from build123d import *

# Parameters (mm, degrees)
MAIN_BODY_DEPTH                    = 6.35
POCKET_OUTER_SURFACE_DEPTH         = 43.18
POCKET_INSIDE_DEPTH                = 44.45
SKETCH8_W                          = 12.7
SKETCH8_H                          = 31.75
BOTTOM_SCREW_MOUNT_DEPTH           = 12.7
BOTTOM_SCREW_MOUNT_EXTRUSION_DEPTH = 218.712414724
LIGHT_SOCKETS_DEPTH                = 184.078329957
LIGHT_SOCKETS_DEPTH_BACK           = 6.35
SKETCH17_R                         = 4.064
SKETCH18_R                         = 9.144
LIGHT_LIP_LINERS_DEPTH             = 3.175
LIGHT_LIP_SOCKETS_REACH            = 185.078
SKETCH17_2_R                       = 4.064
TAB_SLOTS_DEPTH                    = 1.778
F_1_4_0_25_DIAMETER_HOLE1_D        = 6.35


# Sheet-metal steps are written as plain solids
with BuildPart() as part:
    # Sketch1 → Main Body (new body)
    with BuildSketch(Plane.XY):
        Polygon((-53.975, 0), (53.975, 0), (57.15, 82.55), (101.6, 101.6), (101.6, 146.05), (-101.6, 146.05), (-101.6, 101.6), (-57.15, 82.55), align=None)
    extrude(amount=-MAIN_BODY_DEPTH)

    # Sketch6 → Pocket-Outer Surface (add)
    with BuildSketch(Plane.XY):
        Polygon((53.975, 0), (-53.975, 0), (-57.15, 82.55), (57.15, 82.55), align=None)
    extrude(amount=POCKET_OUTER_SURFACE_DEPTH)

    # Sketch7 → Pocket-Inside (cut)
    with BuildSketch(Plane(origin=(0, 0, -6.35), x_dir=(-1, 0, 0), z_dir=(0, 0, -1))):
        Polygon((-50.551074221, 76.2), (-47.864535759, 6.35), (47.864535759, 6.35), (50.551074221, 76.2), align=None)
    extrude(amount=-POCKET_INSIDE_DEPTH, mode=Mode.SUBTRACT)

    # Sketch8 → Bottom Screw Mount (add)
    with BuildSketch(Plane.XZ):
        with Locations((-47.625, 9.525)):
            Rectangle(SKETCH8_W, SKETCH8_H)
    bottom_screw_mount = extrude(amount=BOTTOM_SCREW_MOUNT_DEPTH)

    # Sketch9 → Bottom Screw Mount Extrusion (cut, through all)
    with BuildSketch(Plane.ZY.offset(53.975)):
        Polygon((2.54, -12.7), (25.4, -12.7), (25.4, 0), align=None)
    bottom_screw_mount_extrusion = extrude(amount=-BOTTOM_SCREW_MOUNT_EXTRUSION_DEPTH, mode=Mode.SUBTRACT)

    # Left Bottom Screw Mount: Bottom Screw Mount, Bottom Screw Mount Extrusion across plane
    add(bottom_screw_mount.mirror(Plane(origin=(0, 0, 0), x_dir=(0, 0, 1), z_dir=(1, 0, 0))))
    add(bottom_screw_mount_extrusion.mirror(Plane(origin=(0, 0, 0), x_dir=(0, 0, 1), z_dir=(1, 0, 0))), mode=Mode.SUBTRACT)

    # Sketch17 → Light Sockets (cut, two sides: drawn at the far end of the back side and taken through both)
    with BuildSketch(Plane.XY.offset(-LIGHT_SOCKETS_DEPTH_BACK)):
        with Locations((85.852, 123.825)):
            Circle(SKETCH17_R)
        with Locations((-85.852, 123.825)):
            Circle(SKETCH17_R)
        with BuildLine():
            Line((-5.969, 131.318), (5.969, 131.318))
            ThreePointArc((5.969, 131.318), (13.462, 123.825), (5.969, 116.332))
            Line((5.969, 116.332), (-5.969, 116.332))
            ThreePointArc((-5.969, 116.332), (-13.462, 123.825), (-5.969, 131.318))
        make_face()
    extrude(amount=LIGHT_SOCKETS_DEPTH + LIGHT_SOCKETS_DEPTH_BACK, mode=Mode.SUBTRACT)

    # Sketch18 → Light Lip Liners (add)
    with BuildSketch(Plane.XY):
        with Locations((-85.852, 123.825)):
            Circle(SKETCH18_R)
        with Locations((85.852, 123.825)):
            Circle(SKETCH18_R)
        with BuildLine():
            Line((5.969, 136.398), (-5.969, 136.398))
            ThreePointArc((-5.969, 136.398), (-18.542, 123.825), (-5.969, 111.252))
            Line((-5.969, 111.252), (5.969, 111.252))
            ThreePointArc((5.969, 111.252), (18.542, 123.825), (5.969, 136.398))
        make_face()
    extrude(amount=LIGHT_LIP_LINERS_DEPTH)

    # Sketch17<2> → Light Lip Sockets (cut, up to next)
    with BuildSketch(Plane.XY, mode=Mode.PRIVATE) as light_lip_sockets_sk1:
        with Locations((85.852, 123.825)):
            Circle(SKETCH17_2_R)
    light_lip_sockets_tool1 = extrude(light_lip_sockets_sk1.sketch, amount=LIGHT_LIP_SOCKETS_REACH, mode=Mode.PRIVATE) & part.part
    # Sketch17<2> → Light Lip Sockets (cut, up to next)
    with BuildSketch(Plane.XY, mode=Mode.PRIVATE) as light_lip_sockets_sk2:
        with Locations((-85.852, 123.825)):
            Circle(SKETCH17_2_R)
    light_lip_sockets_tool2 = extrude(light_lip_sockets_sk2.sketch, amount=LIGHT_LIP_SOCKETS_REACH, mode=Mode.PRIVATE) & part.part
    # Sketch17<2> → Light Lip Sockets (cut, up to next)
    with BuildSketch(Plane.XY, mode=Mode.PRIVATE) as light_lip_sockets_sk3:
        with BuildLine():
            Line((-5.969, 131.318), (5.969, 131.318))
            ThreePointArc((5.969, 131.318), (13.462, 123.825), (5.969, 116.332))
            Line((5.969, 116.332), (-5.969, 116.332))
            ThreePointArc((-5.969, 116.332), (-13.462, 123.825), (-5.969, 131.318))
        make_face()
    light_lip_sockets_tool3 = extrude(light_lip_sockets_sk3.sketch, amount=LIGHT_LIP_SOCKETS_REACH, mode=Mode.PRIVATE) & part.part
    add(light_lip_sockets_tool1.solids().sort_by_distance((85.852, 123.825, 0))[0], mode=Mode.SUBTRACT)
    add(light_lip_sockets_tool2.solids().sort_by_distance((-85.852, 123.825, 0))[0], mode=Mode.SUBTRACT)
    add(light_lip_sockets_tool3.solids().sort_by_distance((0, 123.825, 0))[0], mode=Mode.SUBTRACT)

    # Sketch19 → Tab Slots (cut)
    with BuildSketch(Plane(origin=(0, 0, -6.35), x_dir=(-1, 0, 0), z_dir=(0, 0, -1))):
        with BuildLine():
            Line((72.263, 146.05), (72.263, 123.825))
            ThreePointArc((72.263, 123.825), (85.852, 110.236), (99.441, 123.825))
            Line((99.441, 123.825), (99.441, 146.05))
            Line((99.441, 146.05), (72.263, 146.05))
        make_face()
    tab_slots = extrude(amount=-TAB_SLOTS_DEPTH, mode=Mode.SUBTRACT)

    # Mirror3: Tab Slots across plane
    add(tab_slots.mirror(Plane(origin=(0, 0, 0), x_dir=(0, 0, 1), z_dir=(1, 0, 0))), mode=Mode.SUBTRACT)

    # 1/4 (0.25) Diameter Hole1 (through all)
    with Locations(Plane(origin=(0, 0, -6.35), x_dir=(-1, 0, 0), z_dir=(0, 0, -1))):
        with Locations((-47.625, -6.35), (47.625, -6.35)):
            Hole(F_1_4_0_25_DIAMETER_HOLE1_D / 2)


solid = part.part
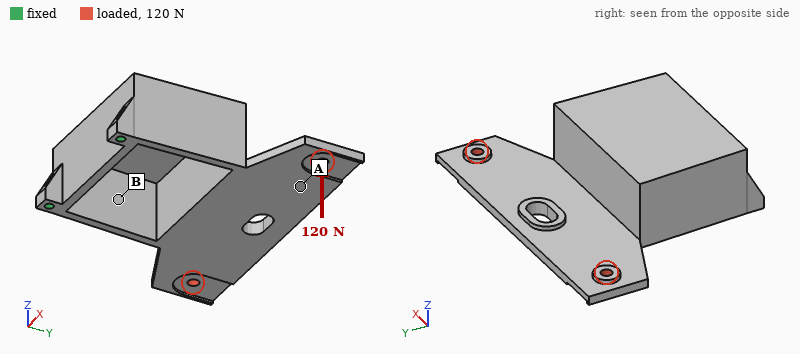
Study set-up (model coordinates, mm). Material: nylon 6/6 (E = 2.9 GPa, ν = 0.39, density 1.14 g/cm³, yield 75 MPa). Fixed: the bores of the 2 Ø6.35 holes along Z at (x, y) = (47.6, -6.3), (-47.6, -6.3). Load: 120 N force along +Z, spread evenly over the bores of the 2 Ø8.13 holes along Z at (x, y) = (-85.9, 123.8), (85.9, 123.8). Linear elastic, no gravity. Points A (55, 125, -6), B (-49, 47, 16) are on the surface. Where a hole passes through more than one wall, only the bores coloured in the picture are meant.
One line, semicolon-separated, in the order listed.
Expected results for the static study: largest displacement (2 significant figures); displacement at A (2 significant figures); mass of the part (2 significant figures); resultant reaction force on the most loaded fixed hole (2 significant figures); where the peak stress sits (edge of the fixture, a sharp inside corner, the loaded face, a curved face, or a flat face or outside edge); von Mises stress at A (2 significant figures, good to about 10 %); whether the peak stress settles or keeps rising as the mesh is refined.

2.8 mm; 1.2 mm; 260 g; 63 N; edge of the fixture; 3.4 MPa; keeps rising
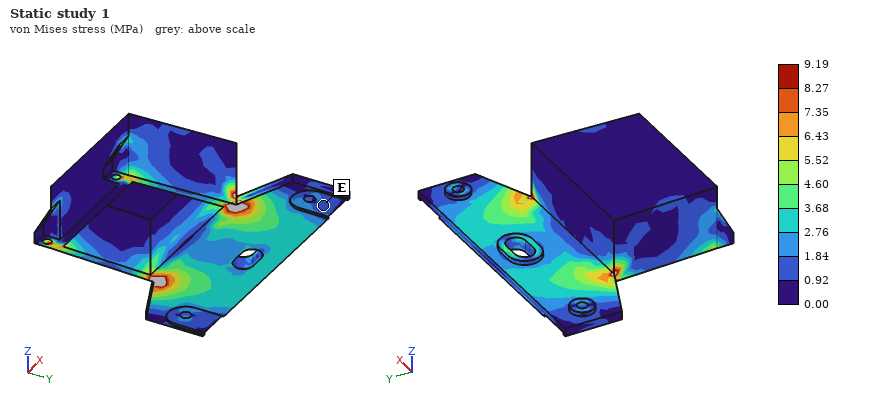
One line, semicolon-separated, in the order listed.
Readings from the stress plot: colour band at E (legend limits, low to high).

0.92 to 1.84 MPa
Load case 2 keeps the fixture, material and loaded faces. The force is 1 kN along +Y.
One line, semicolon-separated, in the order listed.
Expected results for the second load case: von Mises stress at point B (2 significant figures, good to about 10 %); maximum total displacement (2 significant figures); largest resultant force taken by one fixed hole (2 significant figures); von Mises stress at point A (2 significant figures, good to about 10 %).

1.9 MPa; 0.55 mm; 500 N; 1.3 MPa
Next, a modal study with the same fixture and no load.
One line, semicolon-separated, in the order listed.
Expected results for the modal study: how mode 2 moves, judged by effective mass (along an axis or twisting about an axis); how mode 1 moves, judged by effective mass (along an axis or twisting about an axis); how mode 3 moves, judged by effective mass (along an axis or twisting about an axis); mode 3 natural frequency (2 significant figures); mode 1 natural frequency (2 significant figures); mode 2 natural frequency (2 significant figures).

along X; along Z; along X; 360 Hz; 190 Hz; 210 Hz
